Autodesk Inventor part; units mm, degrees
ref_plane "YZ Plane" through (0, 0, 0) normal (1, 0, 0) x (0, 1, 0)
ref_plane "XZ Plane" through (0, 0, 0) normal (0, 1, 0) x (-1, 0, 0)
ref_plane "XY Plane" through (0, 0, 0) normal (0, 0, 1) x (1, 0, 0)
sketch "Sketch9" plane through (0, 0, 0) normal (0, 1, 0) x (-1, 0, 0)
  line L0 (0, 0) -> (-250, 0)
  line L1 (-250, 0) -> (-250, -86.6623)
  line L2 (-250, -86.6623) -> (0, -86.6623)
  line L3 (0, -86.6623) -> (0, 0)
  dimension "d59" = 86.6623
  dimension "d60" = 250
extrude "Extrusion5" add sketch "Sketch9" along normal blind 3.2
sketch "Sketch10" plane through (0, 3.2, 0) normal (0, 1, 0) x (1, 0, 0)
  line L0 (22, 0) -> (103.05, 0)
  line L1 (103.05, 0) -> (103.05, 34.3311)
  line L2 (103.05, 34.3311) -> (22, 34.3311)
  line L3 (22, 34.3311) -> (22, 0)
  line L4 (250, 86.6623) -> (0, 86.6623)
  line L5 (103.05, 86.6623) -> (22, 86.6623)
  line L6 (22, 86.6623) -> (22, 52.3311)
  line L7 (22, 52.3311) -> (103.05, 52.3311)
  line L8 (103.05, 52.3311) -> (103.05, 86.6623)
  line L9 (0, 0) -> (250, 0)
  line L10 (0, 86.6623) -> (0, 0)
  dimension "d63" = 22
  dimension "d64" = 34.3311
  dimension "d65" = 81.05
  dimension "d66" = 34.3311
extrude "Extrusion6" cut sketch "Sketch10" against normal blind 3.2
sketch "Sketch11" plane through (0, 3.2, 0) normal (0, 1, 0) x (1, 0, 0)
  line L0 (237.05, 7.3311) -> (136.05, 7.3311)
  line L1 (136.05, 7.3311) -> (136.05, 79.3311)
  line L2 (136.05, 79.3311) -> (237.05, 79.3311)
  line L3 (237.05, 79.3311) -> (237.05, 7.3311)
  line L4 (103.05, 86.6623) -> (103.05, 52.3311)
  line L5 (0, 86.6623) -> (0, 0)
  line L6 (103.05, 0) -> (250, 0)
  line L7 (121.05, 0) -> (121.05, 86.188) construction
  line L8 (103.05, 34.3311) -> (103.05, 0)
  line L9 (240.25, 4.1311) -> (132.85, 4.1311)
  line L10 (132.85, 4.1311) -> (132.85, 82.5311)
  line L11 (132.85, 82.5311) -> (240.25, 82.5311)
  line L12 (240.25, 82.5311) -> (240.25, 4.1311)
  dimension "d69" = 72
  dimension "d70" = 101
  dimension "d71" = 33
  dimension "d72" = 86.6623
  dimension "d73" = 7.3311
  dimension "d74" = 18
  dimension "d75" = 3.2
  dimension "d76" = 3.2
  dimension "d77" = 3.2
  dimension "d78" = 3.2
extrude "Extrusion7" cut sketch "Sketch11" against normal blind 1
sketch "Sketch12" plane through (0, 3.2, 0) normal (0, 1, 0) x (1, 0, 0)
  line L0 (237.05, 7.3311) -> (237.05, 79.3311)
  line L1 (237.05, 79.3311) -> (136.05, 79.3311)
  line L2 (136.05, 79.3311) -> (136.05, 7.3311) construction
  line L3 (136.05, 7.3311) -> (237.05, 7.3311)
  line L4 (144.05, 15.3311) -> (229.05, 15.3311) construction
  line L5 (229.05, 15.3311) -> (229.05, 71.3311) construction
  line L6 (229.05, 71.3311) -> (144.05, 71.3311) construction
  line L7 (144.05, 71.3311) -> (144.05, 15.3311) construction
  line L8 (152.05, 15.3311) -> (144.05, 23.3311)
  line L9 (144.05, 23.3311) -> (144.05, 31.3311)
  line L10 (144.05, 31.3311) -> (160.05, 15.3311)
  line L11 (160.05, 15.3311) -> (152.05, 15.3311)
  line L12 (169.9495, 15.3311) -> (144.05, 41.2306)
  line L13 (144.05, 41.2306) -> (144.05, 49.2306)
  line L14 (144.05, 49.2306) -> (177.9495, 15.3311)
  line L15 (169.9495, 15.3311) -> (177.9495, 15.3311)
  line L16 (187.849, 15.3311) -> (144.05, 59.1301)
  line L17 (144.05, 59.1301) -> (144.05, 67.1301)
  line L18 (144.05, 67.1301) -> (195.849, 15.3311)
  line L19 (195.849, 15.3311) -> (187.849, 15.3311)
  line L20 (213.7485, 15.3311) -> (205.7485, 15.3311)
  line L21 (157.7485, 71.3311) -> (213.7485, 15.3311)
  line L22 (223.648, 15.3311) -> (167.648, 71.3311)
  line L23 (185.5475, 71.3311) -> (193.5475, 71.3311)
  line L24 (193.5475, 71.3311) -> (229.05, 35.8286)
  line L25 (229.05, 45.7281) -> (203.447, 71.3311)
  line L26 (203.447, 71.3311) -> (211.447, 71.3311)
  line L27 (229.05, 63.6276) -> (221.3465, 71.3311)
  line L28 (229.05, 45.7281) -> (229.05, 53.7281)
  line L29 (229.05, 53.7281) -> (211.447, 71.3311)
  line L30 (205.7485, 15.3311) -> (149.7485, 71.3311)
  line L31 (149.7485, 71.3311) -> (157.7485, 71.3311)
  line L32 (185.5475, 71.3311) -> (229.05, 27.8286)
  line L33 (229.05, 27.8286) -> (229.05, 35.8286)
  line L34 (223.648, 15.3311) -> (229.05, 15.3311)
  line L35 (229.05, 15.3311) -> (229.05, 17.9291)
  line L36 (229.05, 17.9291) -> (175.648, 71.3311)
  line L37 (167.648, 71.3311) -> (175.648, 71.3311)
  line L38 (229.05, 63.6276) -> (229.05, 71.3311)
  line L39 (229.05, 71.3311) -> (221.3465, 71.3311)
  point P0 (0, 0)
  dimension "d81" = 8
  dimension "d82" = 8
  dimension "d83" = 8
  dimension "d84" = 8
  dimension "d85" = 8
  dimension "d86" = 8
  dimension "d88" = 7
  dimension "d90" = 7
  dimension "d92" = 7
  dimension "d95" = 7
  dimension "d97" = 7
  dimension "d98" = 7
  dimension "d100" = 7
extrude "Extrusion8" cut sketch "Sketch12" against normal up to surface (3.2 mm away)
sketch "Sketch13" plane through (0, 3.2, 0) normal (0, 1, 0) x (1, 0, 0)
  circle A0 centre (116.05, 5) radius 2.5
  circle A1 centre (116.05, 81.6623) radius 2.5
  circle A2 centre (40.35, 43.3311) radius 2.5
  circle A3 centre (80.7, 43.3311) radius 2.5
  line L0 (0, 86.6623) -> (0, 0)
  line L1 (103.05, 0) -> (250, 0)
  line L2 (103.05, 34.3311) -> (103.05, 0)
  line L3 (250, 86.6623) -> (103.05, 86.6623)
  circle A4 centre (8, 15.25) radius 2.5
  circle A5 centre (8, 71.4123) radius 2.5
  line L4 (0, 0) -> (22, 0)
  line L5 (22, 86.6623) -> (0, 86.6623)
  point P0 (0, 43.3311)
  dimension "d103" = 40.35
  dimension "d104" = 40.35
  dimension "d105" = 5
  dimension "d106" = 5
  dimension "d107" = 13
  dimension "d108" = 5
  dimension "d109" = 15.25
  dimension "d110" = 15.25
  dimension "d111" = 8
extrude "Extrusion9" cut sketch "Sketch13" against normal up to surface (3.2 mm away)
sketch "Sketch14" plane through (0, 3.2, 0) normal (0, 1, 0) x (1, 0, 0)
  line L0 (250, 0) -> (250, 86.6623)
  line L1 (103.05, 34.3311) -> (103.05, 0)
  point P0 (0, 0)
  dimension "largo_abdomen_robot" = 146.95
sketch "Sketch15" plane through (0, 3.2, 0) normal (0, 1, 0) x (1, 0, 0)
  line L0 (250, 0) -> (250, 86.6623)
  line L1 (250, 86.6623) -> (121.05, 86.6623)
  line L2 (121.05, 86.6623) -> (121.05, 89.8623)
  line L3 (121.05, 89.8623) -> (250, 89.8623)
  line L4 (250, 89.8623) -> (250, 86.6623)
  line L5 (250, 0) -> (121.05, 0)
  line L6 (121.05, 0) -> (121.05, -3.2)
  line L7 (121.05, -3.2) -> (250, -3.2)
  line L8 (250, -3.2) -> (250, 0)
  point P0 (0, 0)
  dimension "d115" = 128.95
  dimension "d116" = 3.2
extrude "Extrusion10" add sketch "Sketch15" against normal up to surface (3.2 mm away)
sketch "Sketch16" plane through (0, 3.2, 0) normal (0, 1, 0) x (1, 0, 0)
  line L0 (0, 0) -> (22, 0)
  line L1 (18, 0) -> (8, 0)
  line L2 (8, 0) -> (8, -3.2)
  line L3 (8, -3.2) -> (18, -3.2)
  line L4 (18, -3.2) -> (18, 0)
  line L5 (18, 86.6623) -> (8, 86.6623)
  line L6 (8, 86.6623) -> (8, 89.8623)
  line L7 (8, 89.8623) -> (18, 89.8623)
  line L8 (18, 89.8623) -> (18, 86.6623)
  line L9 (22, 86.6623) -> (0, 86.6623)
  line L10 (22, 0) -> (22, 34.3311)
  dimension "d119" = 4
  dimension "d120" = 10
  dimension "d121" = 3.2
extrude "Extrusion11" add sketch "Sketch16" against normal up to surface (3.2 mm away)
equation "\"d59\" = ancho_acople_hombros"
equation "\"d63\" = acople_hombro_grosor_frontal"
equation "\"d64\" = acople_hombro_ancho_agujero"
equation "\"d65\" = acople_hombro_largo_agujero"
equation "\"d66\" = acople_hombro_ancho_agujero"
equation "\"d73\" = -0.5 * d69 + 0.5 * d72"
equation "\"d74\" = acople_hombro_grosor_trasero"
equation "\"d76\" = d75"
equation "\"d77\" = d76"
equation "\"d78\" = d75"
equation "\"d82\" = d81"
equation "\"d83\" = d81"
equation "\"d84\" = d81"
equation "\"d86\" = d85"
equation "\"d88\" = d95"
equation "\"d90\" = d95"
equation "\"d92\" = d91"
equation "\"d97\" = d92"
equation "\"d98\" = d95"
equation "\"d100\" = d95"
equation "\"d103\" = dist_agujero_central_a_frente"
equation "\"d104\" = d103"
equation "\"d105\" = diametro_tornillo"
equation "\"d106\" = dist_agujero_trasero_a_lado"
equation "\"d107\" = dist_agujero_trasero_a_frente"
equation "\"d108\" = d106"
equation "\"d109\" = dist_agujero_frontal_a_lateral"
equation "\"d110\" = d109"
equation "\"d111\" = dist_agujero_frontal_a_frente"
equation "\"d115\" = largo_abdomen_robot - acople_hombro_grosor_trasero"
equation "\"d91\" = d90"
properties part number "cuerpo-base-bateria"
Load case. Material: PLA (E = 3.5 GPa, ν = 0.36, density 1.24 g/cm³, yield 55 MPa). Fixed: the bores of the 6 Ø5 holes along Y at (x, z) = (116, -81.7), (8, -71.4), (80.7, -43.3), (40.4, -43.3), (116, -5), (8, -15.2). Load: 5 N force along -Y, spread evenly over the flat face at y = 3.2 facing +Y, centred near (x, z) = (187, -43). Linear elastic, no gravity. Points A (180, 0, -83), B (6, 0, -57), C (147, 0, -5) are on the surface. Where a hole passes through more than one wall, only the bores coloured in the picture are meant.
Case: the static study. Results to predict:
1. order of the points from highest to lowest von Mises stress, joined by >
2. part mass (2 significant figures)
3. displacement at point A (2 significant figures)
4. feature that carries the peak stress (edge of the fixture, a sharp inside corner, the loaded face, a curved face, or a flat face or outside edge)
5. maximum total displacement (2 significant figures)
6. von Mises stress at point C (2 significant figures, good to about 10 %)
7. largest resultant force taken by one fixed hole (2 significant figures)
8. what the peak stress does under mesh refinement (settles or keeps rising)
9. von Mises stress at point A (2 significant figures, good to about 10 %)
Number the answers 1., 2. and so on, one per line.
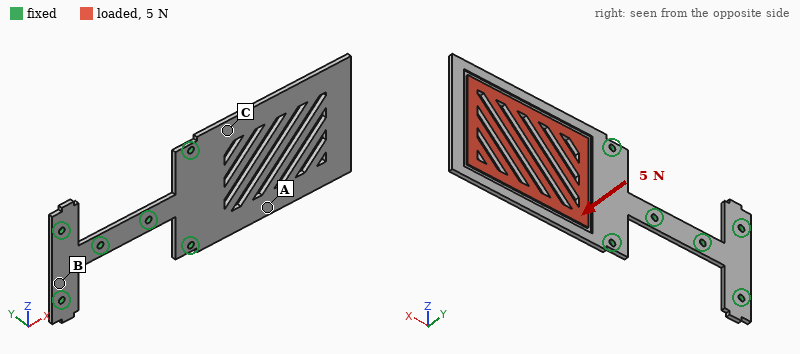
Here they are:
1. C > A > B
2. 57 g
3. 0.94 mm
4. edge of the fixture
5. 2.9 mm
6. 1.8 MPa
7. 3.8 N
8. keeps rising
9. 0.85 MPa
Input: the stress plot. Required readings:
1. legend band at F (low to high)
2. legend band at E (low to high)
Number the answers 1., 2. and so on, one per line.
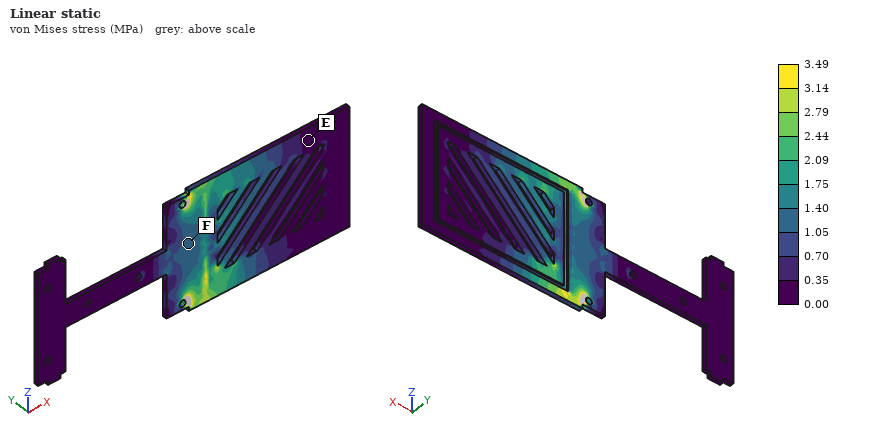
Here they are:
1. 1.05 to 1.40 MPa
2. 0.00 to 0.35 MPa
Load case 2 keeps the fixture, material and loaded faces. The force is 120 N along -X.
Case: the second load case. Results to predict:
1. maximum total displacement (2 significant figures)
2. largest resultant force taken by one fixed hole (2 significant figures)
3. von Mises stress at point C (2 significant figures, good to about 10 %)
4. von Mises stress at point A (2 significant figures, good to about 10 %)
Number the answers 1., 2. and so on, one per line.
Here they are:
1. 2.6 mm
2. 51 N
3. 0.66 MPa
4. 0.83 MPa
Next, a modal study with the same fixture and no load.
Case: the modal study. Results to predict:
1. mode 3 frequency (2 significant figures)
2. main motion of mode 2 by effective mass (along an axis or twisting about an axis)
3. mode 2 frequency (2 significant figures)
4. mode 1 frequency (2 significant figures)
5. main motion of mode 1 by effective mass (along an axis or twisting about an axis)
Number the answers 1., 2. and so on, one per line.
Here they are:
1. 250 Hz
2. twisting about X
3. 120 Hz
4. 41 Hz
5. along Y
